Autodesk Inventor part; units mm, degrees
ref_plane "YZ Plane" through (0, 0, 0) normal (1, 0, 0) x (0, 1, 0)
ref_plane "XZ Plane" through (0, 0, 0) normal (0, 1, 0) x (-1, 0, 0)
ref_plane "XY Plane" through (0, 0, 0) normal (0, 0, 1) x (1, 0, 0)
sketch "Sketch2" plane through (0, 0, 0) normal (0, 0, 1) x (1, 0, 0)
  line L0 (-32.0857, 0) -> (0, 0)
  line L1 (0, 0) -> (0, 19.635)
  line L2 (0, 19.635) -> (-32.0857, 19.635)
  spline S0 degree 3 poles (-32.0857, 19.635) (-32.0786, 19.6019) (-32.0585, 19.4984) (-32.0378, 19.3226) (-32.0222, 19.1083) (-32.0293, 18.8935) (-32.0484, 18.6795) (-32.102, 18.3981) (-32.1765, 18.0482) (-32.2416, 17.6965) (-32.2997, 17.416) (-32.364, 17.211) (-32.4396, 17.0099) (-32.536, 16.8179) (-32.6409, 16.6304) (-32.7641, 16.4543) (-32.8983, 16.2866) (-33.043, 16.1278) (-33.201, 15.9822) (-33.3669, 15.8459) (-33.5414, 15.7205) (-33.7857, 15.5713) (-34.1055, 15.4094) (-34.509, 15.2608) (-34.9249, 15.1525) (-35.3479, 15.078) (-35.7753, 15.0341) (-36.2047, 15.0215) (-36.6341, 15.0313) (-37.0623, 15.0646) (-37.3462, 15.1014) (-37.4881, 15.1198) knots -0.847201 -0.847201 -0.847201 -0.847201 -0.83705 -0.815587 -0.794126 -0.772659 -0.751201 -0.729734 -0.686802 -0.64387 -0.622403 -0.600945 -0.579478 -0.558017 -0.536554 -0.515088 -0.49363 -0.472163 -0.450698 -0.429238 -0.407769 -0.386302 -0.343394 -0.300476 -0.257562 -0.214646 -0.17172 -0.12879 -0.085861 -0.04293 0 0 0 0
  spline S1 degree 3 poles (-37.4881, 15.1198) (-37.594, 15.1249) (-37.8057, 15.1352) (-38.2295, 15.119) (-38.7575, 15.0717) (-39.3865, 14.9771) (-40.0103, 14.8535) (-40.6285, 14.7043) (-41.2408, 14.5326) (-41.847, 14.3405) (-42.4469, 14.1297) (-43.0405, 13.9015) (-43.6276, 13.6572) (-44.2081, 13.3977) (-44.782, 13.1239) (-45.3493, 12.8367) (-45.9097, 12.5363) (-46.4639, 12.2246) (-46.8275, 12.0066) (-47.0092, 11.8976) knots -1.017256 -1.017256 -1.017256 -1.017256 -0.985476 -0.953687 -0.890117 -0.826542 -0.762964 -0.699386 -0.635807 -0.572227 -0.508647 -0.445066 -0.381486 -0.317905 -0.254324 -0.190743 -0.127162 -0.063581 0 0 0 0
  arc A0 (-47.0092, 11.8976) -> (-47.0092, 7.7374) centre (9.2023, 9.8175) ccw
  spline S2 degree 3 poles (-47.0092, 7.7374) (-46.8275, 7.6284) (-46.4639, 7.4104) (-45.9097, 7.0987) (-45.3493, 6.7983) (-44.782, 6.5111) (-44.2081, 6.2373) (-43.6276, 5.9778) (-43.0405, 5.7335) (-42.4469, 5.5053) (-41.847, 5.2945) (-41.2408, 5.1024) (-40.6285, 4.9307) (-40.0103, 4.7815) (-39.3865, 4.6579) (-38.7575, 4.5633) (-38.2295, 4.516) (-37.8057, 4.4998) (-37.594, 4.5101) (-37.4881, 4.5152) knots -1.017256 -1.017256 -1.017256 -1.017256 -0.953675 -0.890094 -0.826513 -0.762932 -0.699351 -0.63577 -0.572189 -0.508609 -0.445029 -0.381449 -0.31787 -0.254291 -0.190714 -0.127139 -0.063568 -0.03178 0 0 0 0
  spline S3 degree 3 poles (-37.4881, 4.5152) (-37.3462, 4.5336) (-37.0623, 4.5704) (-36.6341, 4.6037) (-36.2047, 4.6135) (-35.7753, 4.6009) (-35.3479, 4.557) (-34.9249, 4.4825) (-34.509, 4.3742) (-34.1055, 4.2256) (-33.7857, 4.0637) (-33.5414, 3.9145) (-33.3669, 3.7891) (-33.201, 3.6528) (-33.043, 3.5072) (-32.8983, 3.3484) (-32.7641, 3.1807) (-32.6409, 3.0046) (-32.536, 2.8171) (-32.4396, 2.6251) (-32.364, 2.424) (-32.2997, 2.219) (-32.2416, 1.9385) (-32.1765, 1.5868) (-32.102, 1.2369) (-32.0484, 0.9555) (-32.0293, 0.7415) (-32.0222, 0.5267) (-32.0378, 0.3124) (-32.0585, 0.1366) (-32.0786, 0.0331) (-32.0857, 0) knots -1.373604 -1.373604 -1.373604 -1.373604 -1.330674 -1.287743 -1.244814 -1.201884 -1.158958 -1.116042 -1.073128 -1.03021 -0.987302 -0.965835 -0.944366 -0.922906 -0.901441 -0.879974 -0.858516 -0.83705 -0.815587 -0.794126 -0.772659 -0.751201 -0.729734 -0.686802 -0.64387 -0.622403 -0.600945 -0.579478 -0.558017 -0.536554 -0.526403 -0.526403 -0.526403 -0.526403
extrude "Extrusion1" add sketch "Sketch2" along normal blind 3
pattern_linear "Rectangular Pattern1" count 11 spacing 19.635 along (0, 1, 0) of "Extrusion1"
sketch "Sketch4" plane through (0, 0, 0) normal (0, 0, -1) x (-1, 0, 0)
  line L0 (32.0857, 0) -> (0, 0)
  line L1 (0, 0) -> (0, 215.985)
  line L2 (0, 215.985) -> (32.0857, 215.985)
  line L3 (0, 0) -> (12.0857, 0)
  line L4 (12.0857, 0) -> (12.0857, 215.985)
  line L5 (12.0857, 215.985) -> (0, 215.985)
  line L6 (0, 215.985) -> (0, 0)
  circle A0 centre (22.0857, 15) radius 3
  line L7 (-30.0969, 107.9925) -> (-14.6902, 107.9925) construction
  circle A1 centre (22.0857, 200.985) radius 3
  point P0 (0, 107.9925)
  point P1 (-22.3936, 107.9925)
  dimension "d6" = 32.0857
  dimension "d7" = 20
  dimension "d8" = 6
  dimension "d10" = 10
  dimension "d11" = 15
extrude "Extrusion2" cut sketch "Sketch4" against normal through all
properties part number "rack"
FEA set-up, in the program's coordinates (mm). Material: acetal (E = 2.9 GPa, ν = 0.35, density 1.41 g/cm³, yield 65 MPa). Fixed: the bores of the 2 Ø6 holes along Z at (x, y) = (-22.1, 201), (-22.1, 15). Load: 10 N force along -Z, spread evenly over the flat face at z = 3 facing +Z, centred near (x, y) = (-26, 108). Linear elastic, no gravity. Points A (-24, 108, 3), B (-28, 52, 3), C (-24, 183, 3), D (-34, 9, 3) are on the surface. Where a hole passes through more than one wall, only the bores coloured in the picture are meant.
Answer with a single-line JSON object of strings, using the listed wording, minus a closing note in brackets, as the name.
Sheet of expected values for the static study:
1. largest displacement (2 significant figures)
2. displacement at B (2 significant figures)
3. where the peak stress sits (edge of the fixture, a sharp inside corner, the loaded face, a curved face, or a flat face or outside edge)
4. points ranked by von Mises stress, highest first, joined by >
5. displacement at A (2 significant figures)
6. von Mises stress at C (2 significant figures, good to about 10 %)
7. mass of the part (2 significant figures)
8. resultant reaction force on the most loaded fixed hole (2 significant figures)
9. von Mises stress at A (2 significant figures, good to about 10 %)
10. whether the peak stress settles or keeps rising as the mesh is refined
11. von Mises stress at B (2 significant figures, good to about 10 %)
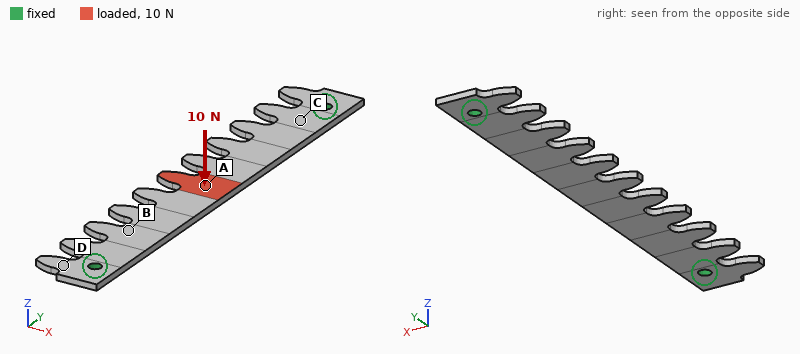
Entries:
{"largest displacement": "2.5 mm", "displacement at B": "0.78 mm", "where the peak stress sits": "edge of the fixture", "points ranked by von Mises stress, highest first, joined by >": "A > C > B > D", "displacement at A": "2.2 mm", "von Mises stress at C": "4.2 MPa", "mass of the part": "25 g", "resultant reaction force on the most loaded fixed hole": "5.0 N", "von Mises stress at A": "6.0 MPa", "whether the peak stress settles or keeps rising as the mesh is refined": "keeps rising", "von Mises stress at B": "1.6 MPa"}
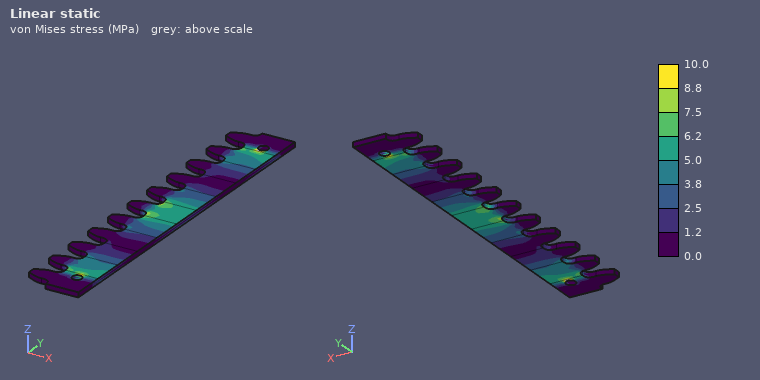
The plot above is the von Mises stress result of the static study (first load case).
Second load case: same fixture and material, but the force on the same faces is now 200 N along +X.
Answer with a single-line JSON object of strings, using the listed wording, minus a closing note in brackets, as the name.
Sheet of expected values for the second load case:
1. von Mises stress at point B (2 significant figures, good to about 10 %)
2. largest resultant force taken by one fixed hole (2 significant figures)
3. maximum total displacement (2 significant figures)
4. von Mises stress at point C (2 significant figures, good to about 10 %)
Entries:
{"von Mises stress at point B": "6.4 MPa", "largest resultant force taken by one fixed hole": "100 N", "maximum total displacement": "2.4 mm", "von Mises stress at point C": "7.7 MPa"}
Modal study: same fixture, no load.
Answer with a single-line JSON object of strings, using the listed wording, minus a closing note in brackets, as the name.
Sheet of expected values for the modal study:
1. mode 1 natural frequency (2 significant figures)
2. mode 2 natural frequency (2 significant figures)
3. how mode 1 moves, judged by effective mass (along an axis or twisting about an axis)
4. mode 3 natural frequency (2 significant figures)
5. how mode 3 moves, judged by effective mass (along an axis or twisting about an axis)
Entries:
{"mode 1 natural frequency": "120 Hz", "mode 2 natural frequency": "320 Hz", "how mode 1 moves, judged by effective mass": "along Z", "mode 3 natural frequency": "390 Hz", "how mode 3 moves, judged by effective mass": "twisting about Y"}
